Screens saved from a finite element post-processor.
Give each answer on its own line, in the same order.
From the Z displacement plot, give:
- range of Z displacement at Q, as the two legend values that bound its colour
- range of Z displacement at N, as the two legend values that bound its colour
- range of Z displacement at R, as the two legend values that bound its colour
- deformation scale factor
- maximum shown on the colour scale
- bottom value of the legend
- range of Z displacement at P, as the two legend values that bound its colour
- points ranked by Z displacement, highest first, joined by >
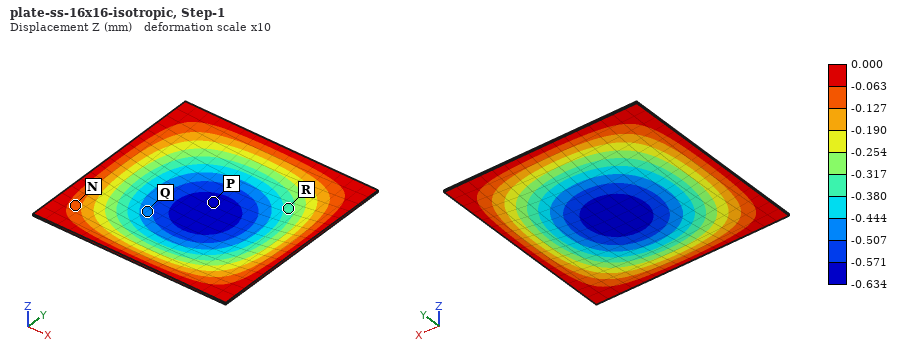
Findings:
-0.507 to -0.444 mm
-0.127 to -0.063 mm
-0.380 to -0.317 mm
10
0.000 mm
-0.634 mm
-0.634 to -0.571 mm
N > R > Q > P
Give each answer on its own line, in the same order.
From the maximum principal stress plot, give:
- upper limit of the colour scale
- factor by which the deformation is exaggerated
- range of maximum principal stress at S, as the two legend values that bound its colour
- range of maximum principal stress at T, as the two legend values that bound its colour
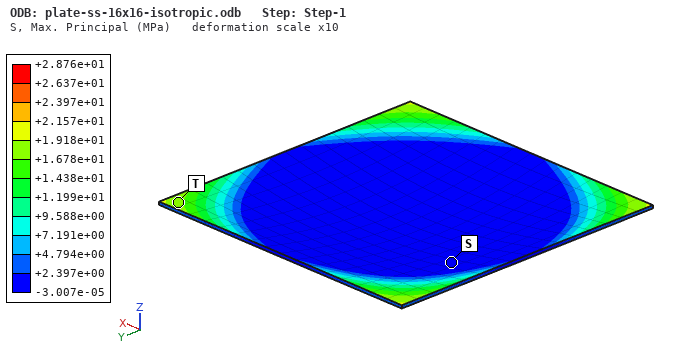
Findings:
+2.876e+01 MPa
10
-3.007e-05 to +2.397e+00 MPa
+1.678e+01 to +1.918e+01 MPa
